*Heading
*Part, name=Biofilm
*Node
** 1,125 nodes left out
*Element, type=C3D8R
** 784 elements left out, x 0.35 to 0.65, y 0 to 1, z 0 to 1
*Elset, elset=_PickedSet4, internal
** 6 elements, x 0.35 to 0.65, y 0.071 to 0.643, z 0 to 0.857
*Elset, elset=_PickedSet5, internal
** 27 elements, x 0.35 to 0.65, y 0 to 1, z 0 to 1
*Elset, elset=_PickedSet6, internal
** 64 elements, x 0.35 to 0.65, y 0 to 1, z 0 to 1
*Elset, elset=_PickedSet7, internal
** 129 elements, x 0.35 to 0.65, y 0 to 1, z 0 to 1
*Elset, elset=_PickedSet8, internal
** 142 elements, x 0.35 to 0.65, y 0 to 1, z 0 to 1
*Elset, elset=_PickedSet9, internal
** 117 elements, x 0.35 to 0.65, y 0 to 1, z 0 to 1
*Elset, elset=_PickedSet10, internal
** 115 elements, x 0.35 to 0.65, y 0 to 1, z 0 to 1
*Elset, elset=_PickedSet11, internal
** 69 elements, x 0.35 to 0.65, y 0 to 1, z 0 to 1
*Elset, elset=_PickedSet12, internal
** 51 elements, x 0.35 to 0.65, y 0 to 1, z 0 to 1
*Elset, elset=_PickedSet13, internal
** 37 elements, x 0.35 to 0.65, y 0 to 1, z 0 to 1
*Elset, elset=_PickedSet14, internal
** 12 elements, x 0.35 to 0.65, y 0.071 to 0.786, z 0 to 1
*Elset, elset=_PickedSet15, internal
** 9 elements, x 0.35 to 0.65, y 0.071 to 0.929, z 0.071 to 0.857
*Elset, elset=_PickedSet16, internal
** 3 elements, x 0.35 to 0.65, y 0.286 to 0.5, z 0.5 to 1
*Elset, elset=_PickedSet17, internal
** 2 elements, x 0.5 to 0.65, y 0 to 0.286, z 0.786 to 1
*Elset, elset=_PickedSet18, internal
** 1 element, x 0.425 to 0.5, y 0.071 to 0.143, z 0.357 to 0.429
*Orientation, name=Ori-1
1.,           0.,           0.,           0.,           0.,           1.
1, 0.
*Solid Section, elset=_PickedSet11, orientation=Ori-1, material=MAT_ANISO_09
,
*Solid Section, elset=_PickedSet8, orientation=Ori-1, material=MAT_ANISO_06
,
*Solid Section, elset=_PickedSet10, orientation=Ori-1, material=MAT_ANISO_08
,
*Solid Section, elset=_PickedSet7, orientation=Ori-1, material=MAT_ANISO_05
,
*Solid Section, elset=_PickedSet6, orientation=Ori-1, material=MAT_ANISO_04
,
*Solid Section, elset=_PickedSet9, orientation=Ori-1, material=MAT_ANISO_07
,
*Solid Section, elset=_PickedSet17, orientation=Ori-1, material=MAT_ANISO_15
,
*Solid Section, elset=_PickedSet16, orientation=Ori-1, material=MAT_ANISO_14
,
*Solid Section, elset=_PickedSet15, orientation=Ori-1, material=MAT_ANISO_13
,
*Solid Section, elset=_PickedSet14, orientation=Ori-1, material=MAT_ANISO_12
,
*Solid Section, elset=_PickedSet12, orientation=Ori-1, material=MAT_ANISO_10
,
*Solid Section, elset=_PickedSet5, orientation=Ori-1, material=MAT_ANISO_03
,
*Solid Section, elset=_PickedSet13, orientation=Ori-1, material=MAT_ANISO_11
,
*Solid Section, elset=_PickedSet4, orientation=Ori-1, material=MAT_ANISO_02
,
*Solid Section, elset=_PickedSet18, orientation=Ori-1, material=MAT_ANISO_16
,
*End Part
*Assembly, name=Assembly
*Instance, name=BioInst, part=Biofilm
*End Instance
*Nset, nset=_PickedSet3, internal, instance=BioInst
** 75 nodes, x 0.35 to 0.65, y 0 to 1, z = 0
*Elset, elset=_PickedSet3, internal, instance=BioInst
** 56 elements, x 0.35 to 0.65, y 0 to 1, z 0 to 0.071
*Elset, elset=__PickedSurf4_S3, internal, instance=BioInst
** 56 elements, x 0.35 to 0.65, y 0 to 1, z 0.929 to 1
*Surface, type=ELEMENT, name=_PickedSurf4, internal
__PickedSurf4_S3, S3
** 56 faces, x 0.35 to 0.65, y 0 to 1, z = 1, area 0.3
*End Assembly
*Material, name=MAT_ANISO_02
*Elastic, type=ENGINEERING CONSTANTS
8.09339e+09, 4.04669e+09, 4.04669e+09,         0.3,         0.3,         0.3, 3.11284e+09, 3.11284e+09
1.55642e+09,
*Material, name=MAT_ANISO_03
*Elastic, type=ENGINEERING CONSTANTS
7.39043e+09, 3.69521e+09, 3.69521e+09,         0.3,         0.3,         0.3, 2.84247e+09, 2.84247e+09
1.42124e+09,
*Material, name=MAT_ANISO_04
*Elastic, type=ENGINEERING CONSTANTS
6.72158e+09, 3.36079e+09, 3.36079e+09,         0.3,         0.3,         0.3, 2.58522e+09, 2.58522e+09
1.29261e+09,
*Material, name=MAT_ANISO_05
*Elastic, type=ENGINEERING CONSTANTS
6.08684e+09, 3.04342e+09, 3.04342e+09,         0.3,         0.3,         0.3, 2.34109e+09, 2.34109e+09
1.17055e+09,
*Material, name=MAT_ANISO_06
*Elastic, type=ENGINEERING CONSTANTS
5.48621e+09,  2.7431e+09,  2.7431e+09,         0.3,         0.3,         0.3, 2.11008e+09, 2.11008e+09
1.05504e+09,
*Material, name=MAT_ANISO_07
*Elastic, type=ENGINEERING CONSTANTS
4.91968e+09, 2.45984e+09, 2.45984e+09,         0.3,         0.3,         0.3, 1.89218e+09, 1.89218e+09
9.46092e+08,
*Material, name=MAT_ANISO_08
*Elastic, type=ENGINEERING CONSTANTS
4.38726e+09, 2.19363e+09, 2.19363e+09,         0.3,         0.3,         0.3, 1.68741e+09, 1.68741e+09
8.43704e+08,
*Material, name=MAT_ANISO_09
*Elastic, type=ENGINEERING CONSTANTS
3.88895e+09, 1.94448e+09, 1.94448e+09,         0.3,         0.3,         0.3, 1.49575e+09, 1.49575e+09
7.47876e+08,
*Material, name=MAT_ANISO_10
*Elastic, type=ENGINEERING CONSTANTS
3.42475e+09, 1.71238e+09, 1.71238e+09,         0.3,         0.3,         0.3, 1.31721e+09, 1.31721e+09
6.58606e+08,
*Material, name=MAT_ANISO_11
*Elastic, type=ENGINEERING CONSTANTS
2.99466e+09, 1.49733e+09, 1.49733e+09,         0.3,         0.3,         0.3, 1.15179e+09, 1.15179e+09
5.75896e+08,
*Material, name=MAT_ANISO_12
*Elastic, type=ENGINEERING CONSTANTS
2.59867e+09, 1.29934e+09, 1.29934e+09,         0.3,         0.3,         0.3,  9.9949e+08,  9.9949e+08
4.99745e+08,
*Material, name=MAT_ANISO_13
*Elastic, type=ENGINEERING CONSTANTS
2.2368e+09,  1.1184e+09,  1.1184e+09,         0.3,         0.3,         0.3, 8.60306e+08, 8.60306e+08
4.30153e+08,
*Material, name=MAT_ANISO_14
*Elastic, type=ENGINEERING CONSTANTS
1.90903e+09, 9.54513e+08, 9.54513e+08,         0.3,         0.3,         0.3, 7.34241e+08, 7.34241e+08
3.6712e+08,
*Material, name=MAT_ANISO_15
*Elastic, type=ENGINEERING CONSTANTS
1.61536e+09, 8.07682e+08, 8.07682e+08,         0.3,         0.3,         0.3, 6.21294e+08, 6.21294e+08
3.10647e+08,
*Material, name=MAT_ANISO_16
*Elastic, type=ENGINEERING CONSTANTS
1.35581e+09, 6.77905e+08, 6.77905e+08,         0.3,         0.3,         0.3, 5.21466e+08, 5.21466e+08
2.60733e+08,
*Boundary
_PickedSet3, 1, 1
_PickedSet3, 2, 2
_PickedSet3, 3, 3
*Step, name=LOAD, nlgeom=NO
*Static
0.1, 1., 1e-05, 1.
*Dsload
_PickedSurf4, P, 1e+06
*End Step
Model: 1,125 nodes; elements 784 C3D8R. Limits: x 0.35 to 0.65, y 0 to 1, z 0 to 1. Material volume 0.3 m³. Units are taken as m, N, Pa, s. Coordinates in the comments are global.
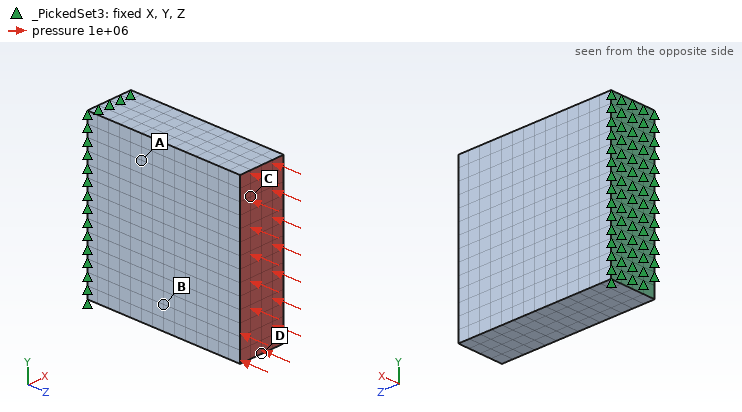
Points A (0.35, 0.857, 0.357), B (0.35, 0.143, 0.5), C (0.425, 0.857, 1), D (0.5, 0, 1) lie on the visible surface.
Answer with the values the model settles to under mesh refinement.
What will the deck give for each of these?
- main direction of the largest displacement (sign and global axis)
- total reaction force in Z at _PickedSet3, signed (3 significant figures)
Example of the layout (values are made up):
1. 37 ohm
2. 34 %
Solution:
1. -Z
2. 3.00e+05 N
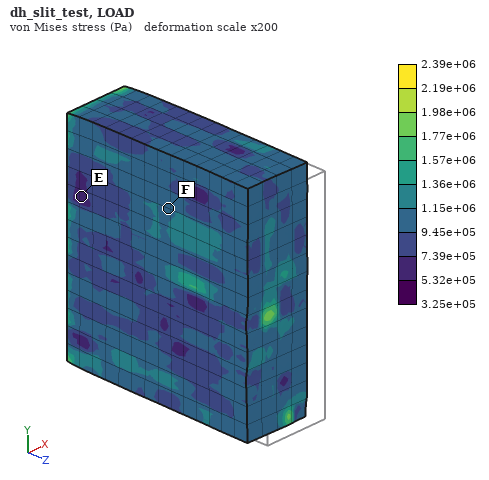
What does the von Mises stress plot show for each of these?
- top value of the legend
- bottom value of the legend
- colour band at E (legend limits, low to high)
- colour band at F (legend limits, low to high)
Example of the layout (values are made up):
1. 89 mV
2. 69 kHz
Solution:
1. 2.39e+06 Pa
2. 3.25e+05 Pa
3. 5.32e+05 to 7.39e+05 Pa
4. 9.45e+05 to 1.15e+06 Pa
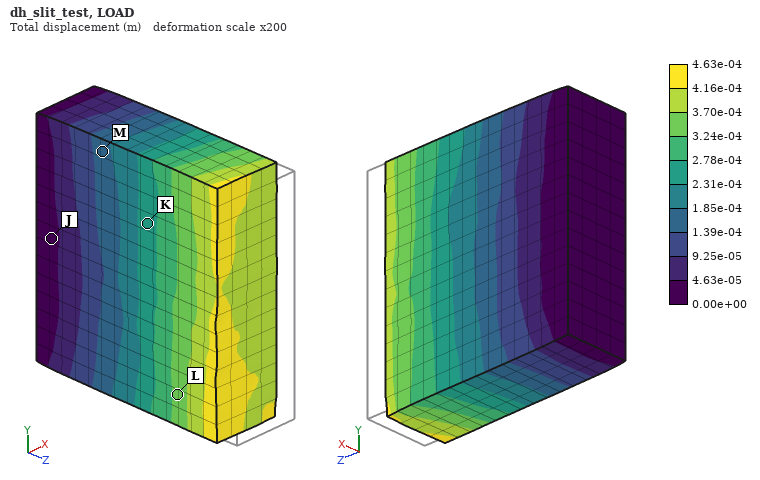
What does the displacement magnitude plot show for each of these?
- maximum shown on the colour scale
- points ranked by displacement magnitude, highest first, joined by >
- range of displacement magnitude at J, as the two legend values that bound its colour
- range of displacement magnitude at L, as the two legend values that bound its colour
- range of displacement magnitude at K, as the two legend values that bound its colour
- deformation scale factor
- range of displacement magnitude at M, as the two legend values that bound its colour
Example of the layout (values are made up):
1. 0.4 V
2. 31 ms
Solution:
1. 4.63e-04 m
2. L > K > M > J
3. 0.00e+00 to 4.63e-05 m
4. 3.24e-04 to 3.70e-04 m
5. 2.31e-04 to 2.78e-04 m
6. 200
7. 1.39e-04 to 1.85e-04 m
